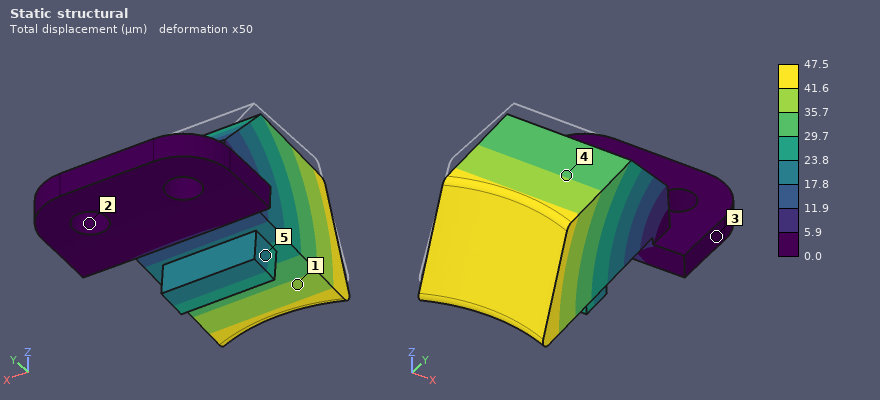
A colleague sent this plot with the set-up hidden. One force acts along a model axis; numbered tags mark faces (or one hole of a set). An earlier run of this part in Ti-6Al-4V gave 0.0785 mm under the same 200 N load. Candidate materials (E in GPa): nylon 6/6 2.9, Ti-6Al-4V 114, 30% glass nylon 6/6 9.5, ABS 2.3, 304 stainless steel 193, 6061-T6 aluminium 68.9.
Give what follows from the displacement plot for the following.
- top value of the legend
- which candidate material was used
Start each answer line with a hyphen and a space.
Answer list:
- 47.5 µm
- 304 stainless steel
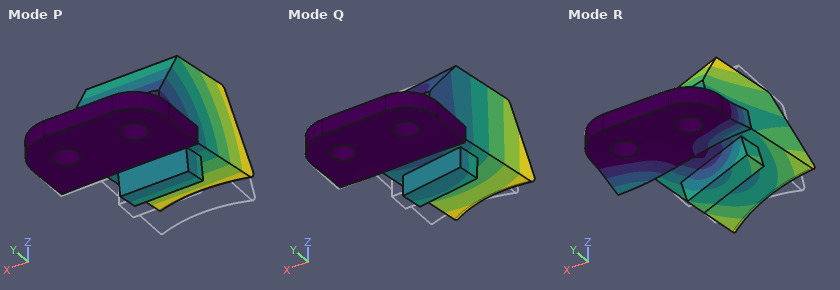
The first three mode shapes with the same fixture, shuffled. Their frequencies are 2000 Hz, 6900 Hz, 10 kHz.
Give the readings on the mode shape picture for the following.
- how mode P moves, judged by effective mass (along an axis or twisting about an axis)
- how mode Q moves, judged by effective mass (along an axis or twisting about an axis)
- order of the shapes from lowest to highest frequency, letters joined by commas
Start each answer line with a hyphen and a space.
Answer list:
- along Z
- along X
- P, Q, R
